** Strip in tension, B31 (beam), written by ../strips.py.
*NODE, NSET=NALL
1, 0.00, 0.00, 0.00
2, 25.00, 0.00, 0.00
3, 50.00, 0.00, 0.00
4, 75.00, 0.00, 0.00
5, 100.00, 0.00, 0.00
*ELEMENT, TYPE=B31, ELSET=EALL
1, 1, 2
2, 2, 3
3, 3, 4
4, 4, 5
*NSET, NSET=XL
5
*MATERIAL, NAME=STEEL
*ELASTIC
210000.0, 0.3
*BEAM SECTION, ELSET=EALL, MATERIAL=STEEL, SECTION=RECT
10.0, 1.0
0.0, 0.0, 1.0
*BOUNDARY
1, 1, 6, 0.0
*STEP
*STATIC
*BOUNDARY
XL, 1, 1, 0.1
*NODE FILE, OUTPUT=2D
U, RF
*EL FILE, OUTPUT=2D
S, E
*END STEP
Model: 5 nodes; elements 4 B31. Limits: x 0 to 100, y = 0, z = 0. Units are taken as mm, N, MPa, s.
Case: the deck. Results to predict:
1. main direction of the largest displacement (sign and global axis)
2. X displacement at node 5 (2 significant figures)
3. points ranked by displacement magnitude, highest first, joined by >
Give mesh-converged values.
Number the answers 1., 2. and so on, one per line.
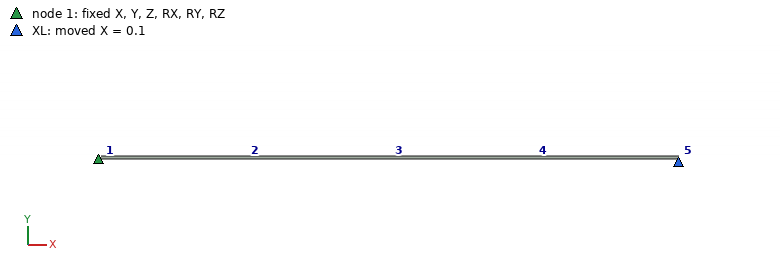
1. +X
2. 0.10 mm
3. node 5 > node 4 > node 3 > node 2 > node 1
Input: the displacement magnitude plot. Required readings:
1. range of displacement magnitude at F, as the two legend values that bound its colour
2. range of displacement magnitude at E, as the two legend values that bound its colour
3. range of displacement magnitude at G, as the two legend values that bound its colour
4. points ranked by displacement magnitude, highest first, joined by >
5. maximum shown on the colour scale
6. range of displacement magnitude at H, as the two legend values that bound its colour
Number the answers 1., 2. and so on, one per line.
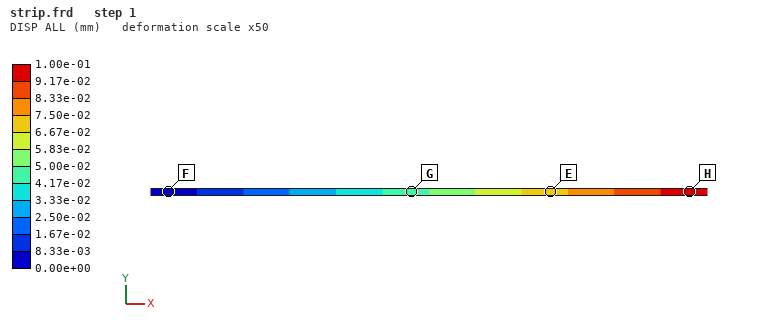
1. 0.00e+00 to 8.33e-03 mm
2. 6.67e-02 to 7.50e-02 mm
3. 4.17e-02 to 5.00e-02 mm
4. H > E > G > F
5. 1.00e-01 mm
6. 9.17e-02 to 1.00e-01 mm
